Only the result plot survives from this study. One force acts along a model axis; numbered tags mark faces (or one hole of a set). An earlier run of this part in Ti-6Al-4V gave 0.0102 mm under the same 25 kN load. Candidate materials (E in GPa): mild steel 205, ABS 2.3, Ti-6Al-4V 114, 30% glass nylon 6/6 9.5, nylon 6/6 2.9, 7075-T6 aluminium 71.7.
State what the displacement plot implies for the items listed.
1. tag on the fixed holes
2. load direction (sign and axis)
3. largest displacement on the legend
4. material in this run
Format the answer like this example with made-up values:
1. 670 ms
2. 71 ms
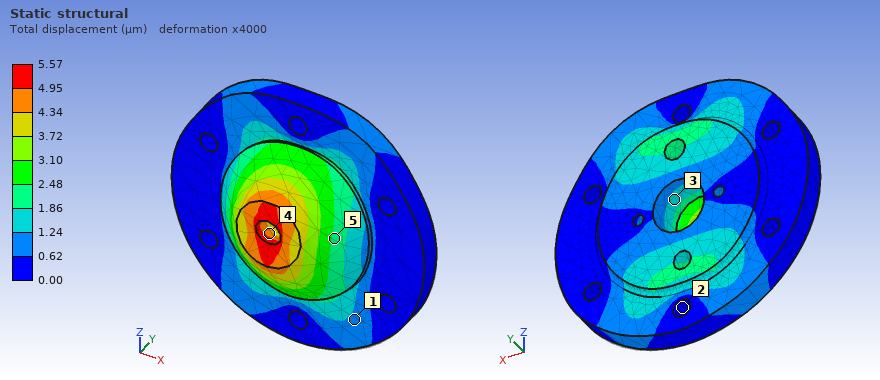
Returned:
1. 2
2. +Z
3. 5.57 µm
4. mild steel
